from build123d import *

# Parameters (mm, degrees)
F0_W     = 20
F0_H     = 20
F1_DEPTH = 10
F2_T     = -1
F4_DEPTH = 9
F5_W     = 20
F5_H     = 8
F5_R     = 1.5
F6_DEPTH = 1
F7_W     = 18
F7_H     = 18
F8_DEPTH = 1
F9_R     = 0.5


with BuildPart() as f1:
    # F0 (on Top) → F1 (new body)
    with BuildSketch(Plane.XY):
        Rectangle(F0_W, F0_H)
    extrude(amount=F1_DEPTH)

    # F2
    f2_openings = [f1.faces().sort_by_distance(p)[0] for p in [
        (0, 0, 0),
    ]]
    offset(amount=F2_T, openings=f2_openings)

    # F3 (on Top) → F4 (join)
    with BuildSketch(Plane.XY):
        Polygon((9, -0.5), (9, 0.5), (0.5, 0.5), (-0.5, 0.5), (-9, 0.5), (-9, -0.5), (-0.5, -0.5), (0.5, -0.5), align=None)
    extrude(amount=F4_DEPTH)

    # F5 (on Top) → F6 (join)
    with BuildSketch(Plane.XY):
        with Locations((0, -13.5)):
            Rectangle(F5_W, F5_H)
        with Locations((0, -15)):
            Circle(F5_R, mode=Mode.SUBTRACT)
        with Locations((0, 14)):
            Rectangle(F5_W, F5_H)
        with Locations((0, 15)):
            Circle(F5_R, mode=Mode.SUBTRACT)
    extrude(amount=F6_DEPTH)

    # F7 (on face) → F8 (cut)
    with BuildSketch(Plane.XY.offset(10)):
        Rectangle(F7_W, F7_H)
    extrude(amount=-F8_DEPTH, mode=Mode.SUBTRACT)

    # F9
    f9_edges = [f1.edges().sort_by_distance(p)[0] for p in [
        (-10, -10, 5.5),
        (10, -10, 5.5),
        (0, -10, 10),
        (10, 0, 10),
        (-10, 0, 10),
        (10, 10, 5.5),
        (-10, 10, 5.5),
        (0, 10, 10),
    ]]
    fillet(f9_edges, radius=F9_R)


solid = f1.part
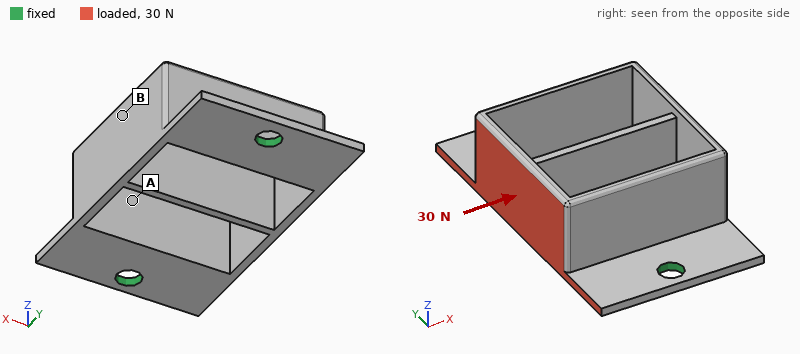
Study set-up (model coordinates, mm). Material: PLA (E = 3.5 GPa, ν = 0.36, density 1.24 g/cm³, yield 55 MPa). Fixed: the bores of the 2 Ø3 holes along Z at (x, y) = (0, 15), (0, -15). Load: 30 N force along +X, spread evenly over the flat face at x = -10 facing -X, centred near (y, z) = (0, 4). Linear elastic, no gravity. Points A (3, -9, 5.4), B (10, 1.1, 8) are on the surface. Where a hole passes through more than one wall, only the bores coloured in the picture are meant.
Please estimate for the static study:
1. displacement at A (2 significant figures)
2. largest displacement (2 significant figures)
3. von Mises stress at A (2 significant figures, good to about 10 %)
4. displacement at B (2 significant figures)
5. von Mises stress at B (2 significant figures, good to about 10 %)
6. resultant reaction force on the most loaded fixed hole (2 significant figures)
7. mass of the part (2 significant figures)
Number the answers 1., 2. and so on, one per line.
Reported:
1. 0.15 mm
2. 0.46 mm
3. 2.4 MPa
4. 0.41 mm
5. 8.1 MPa
6. 15 N
7. 1.5 g
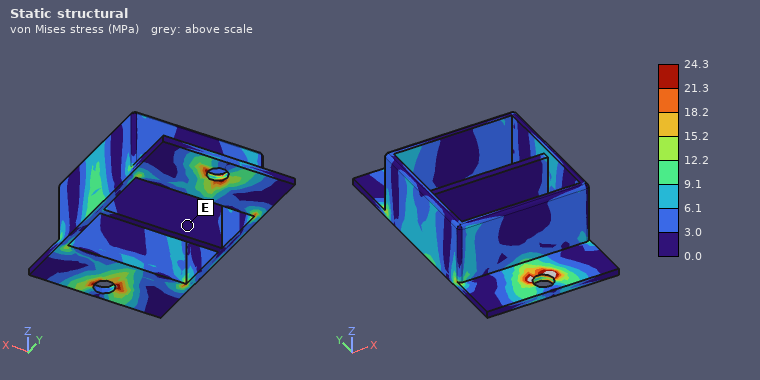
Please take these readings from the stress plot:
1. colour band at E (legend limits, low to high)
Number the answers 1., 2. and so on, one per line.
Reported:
1. 0.0 to 3.0 MPa
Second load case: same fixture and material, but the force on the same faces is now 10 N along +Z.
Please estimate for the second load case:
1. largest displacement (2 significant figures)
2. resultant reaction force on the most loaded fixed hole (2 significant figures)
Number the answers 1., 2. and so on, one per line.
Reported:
1. 0.31 mm
2. 5.6 N
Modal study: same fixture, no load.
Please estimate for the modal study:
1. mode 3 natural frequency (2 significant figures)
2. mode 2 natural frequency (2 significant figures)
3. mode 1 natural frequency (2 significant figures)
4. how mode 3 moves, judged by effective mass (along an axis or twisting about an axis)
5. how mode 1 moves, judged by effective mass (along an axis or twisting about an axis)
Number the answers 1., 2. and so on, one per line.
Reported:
1. 2700 Hz
2. 2500 Hz
3. 1100 Hz
4. along Z
5. along X
